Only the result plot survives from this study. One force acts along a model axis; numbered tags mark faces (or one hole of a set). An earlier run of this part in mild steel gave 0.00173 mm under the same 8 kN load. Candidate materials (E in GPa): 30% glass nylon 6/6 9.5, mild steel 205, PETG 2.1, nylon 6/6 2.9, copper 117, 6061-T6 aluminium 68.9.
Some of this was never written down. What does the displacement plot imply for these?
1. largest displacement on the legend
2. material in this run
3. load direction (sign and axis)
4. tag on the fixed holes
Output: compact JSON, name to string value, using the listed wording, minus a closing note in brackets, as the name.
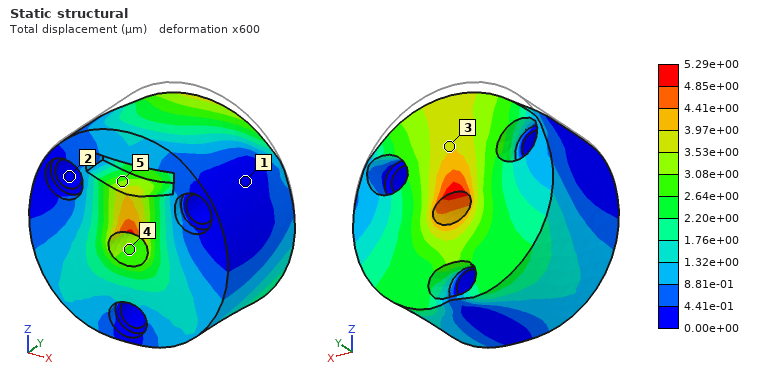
{"largest displacement on the legend": "5.29e+00 µm", "material in this run": "6061-T6 aluminium", "load direction": "-Z", "tag on the fixed holes": "2"}
